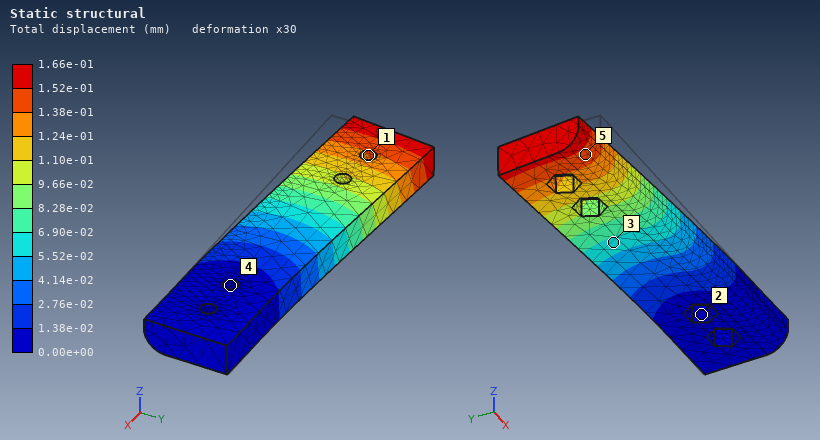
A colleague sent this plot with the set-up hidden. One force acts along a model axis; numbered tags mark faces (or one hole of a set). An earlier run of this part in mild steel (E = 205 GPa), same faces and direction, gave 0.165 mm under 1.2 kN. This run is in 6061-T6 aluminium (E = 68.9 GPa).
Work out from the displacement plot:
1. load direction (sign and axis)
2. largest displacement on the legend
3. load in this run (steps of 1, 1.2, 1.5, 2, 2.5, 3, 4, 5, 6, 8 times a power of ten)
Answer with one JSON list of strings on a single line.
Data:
["+Y", "1.66e-01 mm", "400 N"]
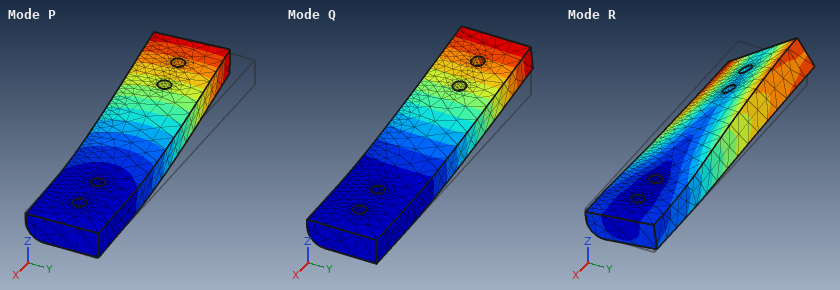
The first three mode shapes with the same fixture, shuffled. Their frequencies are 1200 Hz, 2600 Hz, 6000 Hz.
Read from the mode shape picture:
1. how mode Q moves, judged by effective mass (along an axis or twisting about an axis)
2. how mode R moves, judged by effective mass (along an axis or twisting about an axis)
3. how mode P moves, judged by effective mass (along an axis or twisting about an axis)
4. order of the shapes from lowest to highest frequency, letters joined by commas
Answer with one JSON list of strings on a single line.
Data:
["along Z", "twisting about X", "along Y", "Q, P, R"]
